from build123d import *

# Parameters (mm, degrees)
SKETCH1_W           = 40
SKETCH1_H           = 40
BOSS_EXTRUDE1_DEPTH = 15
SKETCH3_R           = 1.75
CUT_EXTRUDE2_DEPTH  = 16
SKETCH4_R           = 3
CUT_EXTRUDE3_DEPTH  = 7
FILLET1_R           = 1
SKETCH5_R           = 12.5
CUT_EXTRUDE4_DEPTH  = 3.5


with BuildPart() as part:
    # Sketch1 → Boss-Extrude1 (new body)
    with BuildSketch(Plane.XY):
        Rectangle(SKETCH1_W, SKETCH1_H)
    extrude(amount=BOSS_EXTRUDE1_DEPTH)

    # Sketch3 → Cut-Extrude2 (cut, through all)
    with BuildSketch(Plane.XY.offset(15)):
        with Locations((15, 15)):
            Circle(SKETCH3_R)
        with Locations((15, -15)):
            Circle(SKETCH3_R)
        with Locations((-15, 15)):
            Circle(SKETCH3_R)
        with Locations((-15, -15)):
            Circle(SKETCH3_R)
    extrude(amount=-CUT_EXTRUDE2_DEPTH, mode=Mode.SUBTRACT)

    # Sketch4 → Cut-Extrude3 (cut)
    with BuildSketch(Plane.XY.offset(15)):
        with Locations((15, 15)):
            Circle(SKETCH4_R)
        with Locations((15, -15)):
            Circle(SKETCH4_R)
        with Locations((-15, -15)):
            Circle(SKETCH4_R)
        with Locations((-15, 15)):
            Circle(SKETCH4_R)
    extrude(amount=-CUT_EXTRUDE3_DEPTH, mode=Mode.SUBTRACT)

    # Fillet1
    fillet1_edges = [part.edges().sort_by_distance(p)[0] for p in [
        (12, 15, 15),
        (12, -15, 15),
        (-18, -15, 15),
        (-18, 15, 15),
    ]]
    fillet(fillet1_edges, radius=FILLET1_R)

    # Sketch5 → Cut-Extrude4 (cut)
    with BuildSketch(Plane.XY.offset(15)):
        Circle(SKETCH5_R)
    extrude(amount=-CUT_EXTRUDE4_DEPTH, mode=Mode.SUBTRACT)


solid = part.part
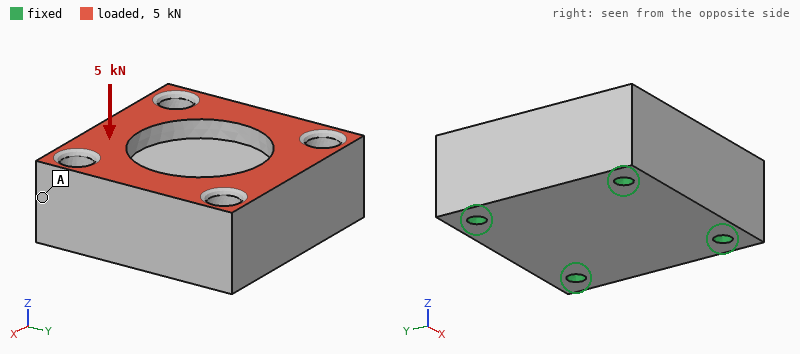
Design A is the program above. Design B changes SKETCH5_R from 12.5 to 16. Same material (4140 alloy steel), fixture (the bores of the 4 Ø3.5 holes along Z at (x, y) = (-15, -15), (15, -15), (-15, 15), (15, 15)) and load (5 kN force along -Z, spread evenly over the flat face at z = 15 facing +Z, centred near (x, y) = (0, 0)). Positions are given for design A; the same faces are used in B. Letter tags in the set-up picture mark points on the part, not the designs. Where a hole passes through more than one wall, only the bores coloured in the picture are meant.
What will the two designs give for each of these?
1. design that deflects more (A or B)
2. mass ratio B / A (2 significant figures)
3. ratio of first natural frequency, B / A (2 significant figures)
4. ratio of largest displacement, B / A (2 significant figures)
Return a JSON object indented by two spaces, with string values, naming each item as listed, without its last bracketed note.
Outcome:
{
  "design that deflects more": "B",
  "mass ratio B / A": "0.95",
  "ratio of first natural frequency, B / A": "1.00",
  "ratio of largest displacement, B / A": "1.2"
}
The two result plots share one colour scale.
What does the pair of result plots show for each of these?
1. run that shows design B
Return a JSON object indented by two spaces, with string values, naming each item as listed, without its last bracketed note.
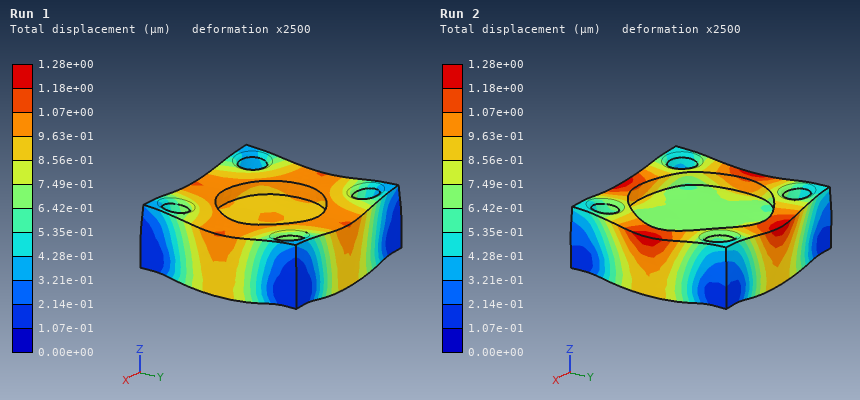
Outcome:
{
  "run that shows design B": "Run 2"
}
